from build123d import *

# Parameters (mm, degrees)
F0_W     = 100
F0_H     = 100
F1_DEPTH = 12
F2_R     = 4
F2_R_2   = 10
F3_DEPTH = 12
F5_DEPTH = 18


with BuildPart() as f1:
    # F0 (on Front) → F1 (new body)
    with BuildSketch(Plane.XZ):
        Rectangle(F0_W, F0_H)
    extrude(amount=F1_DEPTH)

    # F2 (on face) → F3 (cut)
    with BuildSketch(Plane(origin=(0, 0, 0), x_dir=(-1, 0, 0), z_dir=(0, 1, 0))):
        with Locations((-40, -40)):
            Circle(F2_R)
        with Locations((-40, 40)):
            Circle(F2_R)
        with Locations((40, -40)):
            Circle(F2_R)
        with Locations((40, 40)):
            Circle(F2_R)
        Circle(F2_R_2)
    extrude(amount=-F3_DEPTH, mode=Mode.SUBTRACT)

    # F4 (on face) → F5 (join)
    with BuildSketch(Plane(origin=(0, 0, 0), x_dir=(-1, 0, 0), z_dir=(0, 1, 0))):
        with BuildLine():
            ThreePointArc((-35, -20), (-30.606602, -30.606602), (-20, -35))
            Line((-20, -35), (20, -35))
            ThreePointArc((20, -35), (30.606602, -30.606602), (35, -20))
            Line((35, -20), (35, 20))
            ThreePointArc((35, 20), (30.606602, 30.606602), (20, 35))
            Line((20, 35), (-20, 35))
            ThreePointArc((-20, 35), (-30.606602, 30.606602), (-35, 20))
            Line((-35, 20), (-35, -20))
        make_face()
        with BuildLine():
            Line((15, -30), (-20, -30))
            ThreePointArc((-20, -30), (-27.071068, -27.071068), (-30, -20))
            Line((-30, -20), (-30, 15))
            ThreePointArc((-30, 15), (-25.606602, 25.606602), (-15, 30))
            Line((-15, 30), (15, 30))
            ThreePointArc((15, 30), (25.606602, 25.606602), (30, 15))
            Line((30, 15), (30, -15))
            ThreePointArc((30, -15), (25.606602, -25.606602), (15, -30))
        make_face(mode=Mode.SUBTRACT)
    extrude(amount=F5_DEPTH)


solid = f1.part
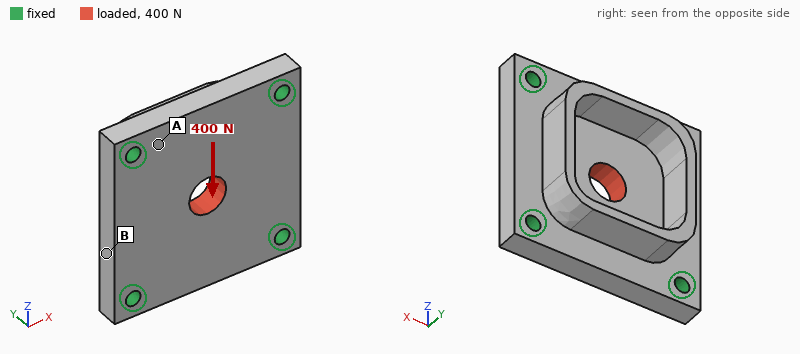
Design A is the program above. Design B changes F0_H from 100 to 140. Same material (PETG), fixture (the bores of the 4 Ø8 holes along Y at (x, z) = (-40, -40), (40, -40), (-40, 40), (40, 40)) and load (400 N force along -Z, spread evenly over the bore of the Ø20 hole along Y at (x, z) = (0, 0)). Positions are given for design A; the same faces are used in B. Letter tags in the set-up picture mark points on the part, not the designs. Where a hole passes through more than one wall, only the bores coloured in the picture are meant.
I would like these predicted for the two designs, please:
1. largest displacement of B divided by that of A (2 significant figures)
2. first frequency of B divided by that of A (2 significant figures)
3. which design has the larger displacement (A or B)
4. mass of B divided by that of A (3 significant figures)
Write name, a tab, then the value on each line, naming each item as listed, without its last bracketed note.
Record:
largest displacement of B divided by that of A	0.85
first frequency of B divided by that of A	0.98
which design has the larger displacement	A
mass of B divided by that of A	1.35
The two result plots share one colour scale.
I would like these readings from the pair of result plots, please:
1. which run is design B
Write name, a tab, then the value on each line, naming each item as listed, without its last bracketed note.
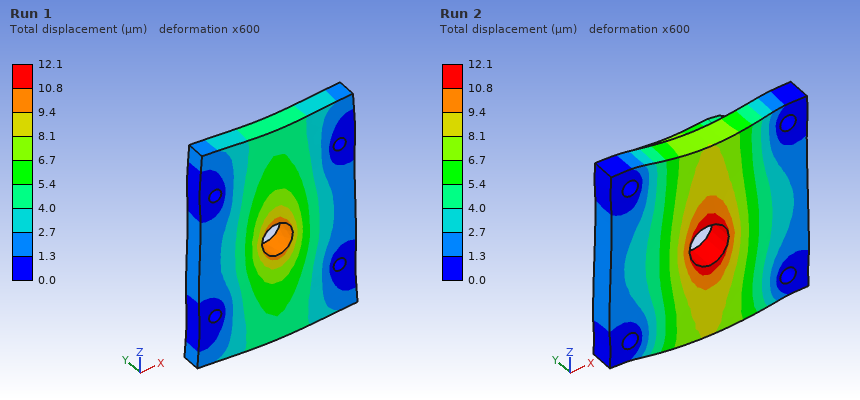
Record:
which run is design B	Run 1
